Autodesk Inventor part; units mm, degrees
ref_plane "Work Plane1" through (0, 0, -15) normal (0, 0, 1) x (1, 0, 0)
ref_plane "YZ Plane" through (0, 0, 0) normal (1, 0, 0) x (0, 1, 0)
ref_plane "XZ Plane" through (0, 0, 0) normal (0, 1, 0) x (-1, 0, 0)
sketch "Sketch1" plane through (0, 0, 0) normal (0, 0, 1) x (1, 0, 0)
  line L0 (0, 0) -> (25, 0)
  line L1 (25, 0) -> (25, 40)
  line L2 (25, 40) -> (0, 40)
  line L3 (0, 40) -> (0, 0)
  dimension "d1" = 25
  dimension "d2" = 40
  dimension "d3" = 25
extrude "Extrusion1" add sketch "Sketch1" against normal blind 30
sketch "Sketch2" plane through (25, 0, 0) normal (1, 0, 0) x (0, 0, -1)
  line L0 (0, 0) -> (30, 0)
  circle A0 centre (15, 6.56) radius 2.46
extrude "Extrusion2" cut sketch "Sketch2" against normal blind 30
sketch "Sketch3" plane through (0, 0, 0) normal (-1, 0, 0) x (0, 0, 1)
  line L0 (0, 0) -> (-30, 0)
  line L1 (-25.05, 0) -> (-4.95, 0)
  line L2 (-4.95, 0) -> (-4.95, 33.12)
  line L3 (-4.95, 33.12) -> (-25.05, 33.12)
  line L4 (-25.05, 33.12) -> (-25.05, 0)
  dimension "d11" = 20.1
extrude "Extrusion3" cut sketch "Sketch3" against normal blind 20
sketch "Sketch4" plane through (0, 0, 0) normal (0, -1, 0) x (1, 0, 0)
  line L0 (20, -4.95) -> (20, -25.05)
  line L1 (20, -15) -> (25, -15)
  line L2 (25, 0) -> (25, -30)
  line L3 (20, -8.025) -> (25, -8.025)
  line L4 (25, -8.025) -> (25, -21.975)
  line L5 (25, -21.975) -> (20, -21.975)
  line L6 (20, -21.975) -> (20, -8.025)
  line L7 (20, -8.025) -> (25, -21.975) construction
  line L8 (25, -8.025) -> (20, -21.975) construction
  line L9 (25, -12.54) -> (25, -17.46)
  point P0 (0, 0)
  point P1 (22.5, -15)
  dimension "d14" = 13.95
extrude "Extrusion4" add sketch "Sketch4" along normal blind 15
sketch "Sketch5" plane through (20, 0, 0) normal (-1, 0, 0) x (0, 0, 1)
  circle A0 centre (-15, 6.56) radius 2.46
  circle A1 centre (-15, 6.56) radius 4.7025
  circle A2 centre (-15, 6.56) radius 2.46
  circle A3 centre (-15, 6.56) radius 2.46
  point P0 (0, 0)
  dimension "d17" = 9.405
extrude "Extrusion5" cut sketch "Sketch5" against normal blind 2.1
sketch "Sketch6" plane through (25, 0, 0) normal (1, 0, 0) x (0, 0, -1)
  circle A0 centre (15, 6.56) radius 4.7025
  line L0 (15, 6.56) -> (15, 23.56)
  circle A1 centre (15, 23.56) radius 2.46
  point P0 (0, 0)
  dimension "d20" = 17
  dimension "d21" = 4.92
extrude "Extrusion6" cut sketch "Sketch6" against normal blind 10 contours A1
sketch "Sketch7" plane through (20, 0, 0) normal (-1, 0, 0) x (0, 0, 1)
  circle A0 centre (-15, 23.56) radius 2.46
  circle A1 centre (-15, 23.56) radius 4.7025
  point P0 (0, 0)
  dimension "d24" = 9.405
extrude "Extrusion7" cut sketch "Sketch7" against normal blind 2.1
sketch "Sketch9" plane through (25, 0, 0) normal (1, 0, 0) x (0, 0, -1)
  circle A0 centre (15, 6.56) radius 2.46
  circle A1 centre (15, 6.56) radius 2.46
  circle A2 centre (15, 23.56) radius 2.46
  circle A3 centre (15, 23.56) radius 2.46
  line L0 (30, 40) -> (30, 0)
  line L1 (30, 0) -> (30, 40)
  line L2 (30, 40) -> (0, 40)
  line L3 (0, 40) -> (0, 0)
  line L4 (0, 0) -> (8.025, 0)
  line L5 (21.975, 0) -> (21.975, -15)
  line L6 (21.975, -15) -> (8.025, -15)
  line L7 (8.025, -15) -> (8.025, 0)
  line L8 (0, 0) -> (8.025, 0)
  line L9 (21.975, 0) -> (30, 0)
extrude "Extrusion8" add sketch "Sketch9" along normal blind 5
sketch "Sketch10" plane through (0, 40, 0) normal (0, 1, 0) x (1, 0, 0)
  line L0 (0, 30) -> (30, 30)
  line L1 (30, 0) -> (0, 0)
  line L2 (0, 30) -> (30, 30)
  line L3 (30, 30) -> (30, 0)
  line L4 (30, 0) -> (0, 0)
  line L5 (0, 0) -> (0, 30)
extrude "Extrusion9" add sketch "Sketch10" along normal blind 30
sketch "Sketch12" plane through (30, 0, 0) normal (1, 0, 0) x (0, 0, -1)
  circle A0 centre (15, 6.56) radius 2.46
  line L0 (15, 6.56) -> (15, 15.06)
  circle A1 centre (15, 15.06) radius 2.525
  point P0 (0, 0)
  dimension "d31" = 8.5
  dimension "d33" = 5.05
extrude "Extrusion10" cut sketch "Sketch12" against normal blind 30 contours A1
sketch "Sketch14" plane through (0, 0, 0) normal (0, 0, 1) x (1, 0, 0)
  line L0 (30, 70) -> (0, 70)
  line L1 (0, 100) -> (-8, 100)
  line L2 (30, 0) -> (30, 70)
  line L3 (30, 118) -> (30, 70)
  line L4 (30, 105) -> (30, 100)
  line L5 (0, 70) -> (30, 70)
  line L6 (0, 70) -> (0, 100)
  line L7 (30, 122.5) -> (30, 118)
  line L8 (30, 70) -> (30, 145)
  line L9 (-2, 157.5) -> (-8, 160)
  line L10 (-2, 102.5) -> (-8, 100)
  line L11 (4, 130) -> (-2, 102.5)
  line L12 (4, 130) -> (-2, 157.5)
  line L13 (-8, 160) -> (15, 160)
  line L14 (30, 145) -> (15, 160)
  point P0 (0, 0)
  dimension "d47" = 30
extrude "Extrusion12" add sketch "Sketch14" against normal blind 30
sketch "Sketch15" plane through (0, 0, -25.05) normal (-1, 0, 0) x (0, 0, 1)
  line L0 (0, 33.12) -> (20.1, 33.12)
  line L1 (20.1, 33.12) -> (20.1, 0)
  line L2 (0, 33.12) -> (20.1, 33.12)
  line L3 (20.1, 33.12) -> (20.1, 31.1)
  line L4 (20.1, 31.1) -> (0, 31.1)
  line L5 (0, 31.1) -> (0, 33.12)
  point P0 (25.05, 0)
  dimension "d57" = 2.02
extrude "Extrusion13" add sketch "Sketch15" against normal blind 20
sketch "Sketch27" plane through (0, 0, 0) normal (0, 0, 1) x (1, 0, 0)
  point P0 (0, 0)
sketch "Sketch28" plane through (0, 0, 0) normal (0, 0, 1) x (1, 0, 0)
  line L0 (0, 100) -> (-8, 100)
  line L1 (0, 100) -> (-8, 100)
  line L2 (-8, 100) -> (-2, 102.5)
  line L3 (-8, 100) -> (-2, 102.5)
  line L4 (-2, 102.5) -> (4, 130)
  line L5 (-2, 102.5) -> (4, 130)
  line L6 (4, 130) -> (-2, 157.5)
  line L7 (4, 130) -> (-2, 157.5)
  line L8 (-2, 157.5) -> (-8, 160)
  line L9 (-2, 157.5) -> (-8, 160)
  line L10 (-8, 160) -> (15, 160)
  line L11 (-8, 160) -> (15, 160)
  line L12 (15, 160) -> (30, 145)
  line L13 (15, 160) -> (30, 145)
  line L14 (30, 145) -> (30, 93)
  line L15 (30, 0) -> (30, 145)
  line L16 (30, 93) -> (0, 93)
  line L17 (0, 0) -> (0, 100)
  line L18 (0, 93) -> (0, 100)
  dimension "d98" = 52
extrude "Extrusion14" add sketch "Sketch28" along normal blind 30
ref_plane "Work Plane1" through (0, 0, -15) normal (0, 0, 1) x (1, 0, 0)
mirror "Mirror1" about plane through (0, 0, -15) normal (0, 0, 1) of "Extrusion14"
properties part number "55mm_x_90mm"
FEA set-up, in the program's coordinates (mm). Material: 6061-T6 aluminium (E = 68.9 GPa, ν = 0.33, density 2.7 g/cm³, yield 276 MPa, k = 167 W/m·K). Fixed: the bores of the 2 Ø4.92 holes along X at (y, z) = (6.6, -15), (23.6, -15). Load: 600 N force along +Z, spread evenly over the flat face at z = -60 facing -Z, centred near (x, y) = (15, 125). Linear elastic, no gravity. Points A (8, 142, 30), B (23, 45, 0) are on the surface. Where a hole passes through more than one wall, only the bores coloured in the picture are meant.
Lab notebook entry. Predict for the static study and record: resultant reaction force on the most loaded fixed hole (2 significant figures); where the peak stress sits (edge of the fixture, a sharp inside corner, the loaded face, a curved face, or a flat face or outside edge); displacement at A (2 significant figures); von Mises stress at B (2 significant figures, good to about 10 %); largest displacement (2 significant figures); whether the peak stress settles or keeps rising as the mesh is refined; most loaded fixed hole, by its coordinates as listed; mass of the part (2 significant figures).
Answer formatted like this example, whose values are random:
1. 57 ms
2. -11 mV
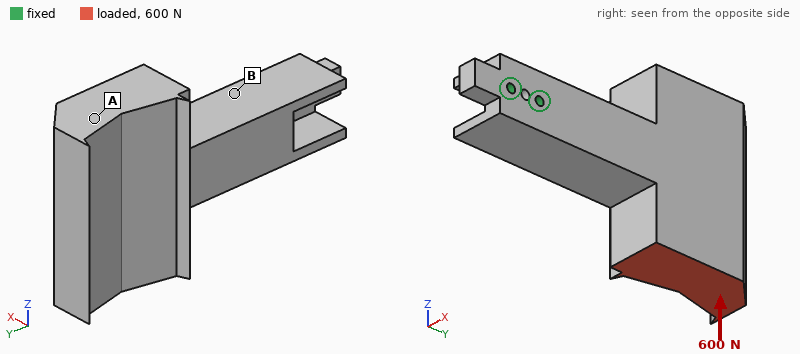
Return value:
1. 3.2 kN
2. edge of the fixture
3. 0.17 mm
4. 13 MPa
5. 0.19 mm
6. keeps rising
7. (23.6, -15)
8. 650 g
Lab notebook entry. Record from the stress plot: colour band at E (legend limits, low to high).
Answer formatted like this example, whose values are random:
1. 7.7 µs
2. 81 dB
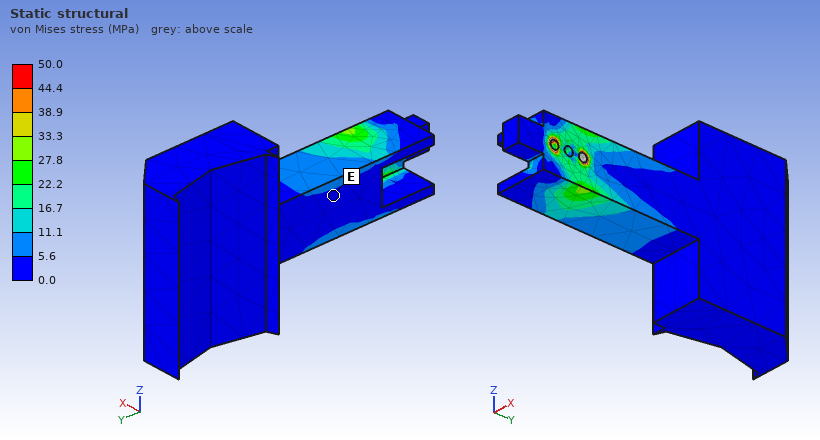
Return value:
1. 0.0 to 5.6 MPa
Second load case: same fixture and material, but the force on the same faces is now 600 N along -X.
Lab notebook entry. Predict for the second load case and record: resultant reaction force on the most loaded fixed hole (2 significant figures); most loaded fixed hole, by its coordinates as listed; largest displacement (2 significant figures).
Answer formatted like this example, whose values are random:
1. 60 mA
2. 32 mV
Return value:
1. 3.0 kN
2. (23.6, -15)
3. 0.34 mm
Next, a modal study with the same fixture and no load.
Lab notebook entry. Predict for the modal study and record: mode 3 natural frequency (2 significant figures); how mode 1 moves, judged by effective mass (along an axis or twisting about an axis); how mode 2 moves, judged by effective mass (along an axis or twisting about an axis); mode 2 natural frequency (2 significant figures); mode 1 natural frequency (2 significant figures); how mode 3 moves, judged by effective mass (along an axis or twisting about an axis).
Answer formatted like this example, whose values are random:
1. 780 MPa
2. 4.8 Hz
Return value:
1. 1000 Hz
2. along X
3. along Z
4. 470 Hz
5. 420 Hz
6. twisting about Y
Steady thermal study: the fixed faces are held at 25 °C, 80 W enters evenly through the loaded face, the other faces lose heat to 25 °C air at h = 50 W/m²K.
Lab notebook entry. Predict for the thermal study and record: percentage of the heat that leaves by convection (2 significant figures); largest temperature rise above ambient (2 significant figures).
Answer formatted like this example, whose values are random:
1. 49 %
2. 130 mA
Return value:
1. 50 %
2. 41 K
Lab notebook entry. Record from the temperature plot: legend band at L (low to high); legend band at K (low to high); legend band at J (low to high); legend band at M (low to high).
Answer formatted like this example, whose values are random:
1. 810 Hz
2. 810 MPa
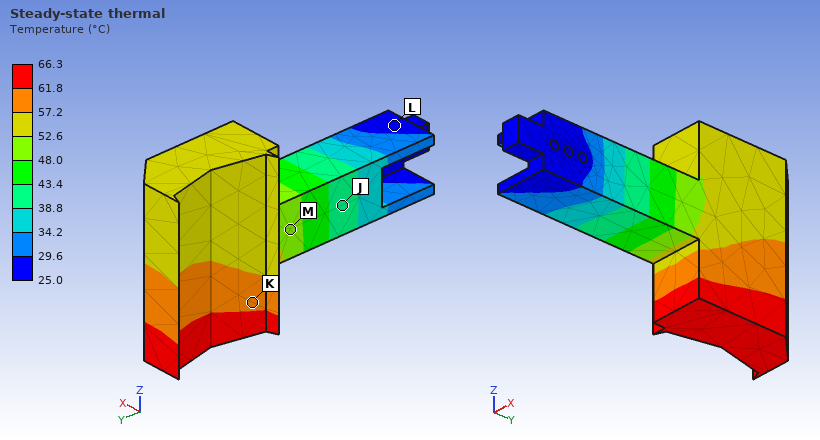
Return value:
1. 25.0 to 29.6 °C
2. 57.2 to 61.8 °C
3. 38.8 to 43.4 °C
4. 48.0 to 52.6 °C
